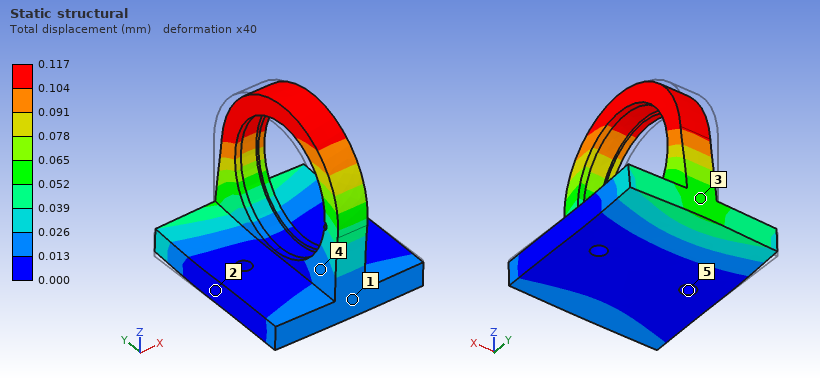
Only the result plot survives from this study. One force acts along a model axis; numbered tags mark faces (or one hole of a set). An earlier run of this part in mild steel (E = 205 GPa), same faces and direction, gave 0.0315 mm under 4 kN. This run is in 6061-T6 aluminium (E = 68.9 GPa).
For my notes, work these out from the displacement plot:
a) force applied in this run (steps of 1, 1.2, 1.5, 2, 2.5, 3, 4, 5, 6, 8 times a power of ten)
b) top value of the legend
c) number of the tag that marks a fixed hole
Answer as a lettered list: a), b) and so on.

a) 5 kN
b) 0.117 mm
c) 5
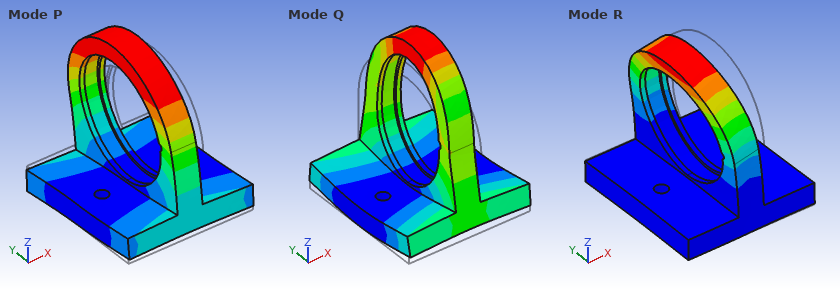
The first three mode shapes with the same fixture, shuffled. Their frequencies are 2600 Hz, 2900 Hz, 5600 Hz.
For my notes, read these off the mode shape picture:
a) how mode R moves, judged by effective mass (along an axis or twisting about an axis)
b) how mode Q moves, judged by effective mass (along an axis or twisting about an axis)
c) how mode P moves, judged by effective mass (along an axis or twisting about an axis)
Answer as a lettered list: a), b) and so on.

a) along X
b) along Z
c) along Y
